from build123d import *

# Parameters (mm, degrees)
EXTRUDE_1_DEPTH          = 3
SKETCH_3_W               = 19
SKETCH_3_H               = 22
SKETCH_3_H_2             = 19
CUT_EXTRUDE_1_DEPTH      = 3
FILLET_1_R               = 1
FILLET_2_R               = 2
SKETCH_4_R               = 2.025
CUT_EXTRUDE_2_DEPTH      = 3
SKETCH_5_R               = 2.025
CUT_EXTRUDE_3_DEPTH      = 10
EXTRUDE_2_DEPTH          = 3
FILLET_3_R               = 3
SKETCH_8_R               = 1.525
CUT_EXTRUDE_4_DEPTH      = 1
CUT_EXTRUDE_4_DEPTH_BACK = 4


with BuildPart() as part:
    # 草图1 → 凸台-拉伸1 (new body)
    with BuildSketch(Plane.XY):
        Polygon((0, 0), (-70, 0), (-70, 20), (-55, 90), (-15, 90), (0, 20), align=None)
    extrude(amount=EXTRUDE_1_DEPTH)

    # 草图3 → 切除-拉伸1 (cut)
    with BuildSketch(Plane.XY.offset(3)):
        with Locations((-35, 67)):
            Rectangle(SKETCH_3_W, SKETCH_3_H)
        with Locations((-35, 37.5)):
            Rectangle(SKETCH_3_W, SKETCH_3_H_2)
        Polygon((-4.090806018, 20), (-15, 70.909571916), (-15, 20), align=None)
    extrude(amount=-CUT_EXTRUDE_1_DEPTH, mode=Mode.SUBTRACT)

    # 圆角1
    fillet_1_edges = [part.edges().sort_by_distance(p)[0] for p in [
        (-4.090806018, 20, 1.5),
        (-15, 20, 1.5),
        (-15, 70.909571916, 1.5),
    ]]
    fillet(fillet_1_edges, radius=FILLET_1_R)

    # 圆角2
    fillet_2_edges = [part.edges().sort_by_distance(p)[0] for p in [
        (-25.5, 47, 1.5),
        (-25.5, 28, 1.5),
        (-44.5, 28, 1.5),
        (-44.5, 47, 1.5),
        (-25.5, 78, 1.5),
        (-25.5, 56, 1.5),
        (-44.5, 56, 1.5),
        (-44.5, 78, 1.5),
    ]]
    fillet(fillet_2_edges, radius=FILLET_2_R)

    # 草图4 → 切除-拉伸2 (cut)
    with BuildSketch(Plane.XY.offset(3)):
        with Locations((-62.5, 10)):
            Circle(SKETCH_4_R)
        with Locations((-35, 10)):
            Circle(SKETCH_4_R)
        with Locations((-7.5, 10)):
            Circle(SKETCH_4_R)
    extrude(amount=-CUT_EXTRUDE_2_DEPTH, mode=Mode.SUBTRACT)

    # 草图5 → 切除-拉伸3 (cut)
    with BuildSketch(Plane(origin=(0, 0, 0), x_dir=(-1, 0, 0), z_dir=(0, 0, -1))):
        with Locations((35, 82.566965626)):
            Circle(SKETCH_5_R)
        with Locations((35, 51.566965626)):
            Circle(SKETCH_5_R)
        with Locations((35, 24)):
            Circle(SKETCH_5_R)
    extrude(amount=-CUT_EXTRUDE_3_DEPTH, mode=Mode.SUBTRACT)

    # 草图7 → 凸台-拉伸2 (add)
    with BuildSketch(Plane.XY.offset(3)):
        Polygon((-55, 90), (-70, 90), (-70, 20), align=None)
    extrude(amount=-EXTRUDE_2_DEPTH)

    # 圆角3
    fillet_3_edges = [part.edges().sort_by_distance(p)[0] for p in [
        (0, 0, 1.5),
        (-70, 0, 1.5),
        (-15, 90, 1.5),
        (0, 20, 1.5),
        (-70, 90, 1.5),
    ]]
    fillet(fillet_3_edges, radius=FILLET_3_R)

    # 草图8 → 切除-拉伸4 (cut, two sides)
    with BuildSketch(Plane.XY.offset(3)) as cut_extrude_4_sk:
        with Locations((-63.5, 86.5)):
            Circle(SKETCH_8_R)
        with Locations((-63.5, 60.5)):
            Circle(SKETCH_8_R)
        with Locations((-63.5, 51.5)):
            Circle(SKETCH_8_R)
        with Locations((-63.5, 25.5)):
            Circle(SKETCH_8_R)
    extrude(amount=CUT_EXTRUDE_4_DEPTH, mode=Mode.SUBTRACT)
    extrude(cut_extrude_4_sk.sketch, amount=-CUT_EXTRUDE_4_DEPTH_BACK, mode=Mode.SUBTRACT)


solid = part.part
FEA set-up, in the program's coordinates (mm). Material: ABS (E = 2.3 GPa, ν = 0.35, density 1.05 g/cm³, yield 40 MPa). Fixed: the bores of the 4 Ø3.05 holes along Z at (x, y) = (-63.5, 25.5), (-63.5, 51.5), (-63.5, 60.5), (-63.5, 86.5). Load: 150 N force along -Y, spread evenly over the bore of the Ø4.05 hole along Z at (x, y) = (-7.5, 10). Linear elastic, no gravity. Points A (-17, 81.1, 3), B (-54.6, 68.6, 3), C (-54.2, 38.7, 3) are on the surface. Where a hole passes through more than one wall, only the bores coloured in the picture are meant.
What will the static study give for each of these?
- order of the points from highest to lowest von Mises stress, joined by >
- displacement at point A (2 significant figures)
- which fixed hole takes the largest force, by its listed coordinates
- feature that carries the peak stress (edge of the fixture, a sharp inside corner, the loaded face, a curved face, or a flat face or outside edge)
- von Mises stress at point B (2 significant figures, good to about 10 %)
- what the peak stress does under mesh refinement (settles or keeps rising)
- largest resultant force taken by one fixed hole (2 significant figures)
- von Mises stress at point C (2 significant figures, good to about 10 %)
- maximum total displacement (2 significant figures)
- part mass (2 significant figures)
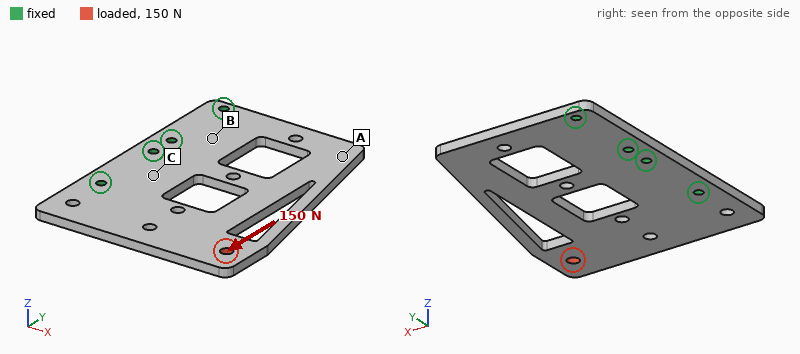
C > B > A
0.24 mm
(-63.5, 25.5)
edge of the fixture
2.5 MPa
keeps rising
150 N
4.0 MPa
0.45 mm
15 g
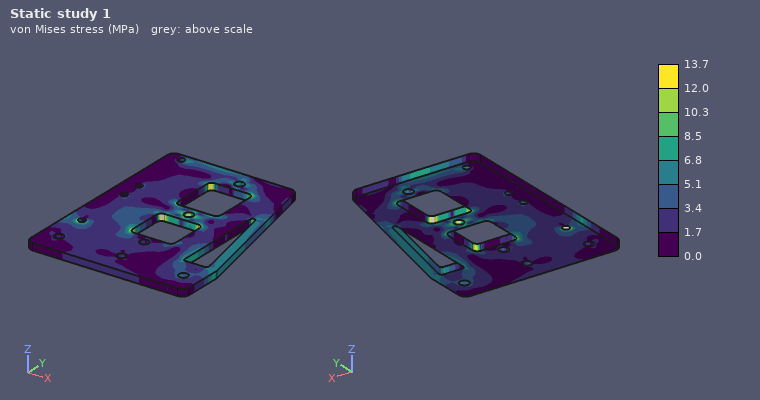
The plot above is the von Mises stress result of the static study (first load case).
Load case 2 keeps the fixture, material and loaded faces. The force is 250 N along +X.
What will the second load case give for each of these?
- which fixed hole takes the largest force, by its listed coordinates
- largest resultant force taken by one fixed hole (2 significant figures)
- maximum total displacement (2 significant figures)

(-63.5, 25.5)
310 N
0.28 mm
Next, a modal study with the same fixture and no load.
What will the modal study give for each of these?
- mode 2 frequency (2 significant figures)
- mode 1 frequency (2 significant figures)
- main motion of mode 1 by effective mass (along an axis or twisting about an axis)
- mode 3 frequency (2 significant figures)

340 Hz
190 Hz
along Z
710 Hz
